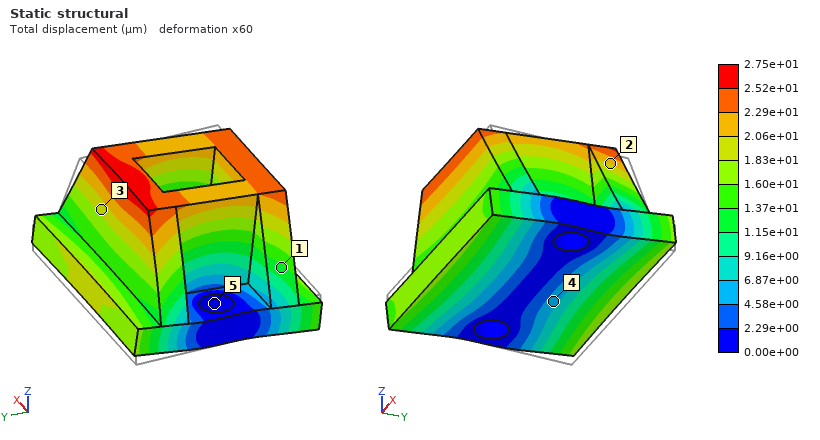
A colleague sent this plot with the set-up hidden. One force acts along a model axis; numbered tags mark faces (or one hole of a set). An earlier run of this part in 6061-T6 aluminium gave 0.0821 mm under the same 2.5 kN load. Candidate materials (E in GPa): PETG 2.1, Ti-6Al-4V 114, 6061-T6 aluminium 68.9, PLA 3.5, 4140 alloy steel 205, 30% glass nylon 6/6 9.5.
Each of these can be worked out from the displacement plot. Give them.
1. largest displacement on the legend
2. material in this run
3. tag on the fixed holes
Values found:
2.75e+01 µm
4140 alloy steel
5
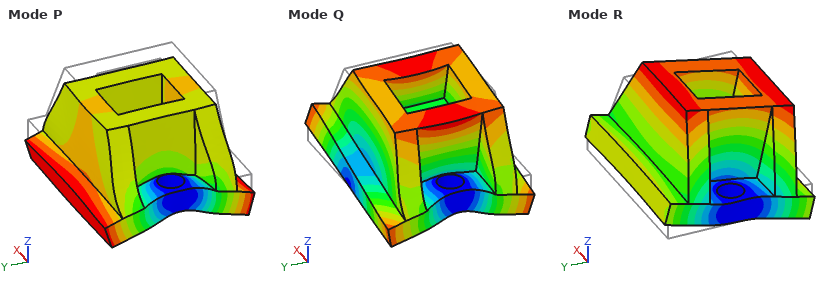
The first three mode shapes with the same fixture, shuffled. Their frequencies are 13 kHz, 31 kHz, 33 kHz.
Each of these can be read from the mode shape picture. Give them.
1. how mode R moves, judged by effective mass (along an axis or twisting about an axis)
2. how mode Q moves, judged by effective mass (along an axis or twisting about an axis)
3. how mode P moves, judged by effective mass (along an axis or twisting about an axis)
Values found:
along Y
along X
along Z
